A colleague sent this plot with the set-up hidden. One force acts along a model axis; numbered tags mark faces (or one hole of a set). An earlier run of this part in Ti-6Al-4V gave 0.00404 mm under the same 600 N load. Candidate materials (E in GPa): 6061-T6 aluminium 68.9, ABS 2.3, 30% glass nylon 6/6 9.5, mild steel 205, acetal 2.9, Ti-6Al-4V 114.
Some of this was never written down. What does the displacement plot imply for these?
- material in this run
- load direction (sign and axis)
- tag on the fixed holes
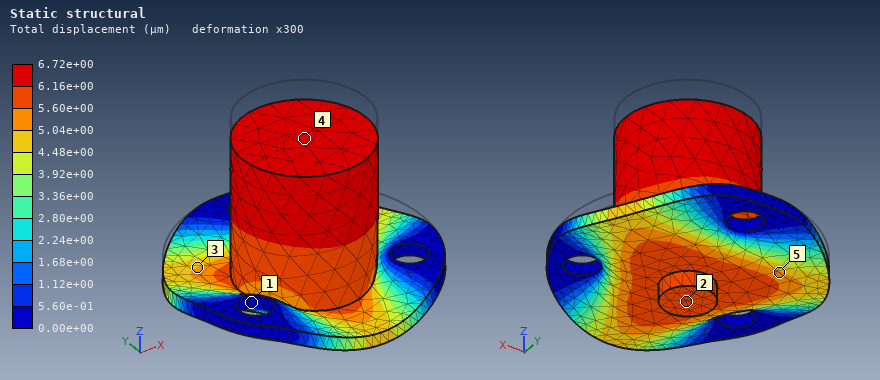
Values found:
6061-T6 aluminium
-Z
1
